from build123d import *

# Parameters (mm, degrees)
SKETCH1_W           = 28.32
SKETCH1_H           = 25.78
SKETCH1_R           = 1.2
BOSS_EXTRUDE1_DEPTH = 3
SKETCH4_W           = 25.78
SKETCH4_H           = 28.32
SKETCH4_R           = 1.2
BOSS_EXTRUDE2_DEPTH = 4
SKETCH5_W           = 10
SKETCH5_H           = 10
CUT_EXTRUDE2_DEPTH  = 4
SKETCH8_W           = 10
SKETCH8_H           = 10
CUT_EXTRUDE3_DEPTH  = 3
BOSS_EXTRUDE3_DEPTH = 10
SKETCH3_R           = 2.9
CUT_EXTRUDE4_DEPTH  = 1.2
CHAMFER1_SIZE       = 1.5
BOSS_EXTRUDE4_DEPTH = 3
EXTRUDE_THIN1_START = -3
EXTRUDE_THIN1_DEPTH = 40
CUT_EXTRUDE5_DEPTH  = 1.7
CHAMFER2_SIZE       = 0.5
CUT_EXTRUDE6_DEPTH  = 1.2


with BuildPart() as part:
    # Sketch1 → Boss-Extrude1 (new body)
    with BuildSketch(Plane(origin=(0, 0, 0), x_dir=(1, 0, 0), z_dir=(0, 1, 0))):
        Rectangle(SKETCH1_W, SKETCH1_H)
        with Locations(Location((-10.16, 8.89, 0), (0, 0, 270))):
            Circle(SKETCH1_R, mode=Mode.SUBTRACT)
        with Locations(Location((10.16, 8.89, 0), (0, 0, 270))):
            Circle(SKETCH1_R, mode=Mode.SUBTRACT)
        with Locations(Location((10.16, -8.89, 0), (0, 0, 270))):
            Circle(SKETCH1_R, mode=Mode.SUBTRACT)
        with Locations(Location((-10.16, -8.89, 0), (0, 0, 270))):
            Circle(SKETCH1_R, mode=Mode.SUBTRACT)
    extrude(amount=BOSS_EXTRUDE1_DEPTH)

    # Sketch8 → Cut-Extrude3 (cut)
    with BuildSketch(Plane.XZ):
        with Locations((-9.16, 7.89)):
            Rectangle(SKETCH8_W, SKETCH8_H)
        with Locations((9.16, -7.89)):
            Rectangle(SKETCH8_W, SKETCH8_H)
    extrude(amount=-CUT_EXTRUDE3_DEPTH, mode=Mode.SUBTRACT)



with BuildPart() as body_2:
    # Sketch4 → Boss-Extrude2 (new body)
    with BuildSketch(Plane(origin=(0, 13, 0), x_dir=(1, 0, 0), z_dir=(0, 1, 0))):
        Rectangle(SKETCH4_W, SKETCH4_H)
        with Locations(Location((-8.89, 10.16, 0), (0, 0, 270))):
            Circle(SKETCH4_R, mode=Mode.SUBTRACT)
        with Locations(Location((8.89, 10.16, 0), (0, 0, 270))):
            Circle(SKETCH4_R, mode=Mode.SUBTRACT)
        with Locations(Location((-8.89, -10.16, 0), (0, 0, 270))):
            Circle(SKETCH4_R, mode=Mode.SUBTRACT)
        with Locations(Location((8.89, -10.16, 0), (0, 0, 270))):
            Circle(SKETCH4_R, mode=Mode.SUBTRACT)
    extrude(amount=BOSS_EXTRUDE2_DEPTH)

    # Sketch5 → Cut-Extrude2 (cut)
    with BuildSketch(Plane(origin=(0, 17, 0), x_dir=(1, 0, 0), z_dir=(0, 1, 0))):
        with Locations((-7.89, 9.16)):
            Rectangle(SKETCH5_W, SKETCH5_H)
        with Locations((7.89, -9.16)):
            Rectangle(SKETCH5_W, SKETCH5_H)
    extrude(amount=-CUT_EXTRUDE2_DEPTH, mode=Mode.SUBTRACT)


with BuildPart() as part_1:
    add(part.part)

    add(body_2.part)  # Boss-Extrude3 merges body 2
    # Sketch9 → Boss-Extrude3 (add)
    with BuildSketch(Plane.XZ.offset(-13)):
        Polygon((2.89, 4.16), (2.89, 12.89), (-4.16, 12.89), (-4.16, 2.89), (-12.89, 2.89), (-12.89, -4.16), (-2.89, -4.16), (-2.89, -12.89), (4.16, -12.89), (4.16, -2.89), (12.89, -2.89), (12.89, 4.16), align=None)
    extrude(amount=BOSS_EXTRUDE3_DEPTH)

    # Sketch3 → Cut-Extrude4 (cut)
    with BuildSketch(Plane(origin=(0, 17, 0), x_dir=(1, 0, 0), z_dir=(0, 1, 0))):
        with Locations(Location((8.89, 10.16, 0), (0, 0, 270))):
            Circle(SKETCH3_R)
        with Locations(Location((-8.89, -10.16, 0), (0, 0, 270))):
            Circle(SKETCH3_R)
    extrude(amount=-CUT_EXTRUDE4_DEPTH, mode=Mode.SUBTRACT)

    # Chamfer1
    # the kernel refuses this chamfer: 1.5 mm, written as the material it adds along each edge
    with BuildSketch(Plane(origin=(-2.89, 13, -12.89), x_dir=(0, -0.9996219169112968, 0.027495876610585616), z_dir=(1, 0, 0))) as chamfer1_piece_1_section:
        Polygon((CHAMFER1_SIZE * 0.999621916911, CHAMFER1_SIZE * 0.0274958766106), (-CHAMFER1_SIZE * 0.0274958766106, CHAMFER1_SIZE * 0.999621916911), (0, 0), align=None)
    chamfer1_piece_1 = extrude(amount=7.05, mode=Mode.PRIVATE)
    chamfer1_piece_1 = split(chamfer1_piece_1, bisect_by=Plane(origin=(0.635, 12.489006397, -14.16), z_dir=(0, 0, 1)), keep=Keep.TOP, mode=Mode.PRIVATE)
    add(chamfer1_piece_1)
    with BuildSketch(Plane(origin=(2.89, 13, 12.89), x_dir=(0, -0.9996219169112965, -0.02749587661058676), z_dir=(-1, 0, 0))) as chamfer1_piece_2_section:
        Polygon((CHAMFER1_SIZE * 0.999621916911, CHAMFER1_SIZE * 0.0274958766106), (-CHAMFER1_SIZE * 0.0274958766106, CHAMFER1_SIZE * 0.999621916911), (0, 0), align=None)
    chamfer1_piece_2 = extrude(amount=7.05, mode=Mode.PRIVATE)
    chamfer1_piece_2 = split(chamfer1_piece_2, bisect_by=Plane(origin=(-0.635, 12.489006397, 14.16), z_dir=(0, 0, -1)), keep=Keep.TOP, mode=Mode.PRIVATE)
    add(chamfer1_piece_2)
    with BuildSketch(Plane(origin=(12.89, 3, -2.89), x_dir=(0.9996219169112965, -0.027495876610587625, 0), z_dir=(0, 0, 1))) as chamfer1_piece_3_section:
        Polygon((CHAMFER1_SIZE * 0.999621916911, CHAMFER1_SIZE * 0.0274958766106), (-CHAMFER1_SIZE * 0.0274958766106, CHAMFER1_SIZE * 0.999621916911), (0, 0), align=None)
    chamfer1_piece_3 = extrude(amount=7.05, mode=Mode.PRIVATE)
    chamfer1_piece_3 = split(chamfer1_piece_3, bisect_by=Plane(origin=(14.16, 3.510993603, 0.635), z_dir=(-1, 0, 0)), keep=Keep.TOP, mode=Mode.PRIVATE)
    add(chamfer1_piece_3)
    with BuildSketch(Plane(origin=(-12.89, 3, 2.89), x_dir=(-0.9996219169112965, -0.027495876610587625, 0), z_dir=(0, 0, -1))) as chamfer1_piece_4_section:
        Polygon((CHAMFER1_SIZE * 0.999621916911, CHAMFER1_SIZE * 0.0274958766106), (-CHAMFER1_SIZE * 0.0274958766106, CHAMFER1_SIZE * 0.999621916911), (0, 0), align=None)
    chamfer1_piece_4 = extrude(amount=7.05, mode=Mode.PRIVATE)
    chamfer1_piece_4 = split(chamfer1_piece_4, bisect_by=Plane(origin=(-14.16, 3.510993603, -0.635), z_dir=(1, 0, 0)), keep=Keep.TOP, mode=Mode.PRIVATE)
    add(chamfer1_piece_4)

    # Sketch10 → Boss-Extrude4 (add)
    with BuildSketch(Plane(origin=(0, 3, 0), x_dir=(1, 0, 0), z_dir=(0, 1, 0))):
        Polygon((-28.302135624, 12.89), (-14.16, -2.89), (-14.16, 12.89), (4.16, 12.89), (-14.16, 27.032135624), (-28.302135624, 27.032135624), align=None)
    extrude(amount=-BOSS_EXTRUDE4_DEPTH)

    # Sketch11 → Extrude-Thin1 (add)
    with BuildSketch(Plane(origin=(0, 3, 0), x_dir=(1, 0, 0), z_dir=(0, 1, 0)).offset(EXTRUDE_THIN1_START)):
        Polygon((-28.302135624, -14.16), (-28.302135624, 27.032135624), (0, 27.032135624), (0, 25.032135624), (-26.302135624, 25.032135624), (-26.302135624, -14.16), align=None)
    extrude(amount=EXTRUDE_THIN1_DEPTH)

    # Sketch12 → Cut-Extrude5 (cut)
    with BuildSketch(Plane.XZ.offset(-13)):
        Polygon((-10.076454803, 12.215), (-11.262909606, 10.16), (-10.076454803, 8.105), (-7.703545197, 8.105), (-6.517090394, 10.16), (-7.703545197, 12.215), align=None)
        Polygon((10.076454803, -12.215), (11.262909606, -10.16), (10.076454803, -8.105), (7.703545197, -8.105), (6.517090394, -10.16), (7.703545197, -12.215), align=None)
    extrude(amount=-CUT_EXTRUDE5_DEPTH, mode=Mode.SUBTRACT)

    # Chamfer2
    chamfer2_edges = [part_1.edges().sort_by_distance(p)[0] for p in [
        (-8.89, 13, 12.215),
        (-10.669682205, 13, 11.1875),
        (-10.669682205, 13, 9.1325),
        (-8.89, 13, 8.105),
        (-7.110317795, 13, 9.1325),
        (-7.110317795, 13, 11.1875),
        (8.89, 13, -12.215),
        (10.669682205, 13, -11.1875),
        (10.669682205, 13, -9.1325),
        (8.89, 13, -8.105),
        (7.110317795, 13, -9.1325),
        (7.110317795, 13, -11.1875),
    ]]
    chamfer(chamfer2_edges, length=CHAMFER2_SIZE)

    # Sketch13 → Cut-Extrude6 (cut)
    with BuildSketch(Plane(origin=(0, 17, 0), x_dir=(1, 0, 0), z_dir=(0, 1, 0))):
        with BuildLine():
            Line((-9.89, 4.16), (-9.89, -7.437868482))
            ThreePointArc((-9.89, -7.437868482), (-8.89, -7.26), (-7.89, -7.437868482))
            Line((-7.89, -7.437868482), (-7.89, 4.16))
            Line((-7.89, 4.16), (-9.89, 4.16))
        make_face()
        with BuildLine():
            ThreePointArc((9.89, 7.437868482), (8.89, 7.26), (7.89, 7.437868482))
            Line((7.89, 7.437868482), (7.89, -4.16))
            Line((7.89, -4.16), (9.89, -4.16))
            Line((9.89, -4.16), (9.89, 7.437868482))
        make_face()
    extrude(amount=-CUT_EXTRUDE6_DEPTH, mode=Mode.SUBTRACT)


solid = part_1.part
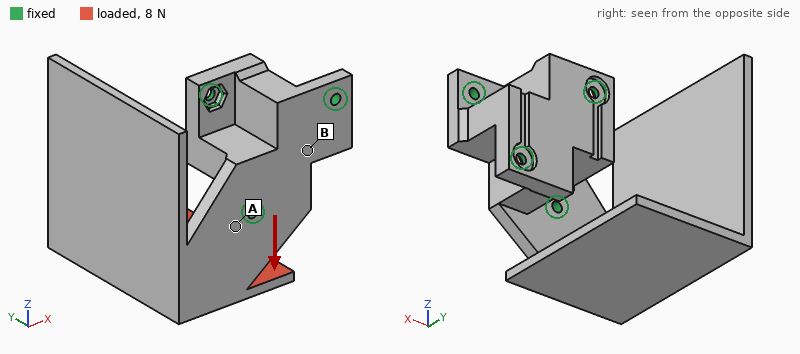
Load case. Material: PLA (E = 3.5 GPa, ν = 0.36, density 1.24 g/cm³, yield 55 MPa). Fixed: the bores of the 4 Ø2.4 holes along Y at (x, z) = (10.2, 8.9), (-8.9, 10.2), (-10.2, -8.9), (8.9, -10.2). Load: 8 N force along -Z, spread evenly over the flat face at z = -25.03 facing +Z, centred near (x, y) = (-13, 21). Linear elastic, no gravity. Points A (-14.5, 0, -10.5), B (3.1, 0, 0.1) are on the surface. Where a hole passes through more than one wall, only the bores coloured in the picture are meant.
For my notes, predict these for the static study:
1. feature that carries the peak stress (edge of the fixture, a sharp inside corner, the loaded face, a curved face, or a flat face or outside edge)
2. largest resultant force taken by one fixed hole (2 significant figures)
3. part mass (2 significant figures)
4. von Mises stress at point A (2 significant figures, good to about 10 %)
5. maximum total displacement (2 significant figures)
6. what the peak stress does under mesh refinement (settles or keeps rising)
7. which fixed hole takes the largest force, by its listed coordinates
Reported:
edge of the fixture
9.5 N
16 g
3.8 MPa
0.80 mm
keeps rising
(-10.2, -8.9)
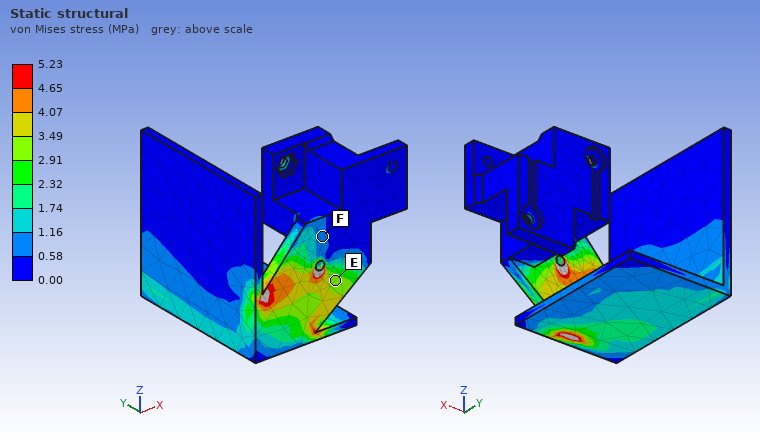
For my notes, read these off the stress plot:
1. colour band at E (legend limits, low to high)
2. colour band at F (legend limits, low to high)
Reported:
2.91 to 3.49 MPa
0.58 to 1.16 MPa
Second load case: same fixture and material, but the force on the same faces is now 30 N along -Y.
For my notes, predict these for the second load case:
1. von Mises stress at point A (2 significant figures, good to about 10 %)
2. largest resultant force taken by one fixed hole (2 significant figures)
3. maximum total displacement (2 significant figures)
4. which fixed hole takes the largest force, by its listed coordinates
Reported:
9.7 MPa
40 N
0.83 mm
(-10.2, -8.9)
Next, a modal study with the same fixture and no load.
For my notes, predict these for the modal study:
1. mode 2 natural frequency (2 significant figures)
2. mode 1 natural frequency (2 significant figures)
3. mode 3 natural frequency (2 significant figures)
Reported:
290 Hz
250 Hz
530 Hz
